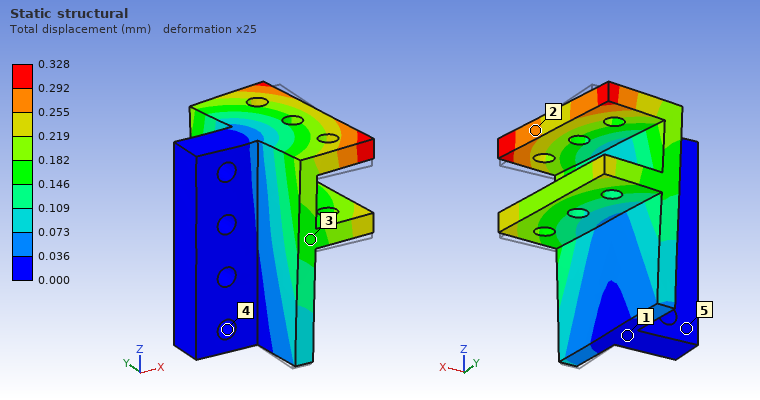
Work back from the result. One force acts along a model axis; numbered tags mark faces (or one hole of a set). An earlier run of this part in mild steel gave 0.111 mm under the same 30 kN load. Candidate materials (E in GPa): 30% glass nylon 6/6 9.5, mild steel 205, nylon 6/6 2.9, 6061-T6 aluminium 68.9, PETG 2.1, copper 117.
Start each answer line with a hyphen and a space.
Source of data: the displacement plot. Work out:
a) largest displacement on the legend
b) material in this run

- 0.328 mm
- 6061-T6 aluminium
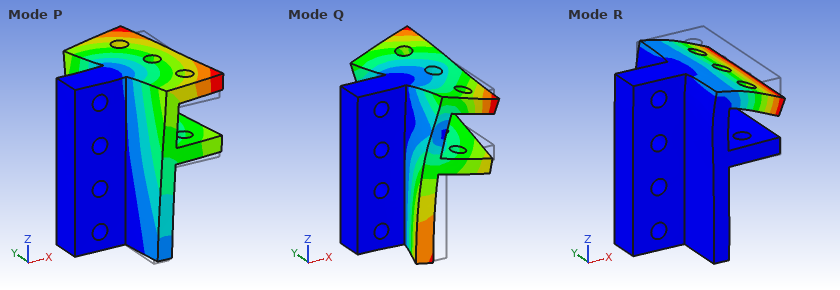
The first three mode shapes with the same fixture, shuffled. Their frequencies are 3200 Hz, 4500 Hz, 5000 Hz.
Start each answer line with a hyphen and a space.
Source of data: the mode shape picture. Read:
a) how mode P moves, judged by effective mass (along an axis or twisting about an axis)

- along Y
